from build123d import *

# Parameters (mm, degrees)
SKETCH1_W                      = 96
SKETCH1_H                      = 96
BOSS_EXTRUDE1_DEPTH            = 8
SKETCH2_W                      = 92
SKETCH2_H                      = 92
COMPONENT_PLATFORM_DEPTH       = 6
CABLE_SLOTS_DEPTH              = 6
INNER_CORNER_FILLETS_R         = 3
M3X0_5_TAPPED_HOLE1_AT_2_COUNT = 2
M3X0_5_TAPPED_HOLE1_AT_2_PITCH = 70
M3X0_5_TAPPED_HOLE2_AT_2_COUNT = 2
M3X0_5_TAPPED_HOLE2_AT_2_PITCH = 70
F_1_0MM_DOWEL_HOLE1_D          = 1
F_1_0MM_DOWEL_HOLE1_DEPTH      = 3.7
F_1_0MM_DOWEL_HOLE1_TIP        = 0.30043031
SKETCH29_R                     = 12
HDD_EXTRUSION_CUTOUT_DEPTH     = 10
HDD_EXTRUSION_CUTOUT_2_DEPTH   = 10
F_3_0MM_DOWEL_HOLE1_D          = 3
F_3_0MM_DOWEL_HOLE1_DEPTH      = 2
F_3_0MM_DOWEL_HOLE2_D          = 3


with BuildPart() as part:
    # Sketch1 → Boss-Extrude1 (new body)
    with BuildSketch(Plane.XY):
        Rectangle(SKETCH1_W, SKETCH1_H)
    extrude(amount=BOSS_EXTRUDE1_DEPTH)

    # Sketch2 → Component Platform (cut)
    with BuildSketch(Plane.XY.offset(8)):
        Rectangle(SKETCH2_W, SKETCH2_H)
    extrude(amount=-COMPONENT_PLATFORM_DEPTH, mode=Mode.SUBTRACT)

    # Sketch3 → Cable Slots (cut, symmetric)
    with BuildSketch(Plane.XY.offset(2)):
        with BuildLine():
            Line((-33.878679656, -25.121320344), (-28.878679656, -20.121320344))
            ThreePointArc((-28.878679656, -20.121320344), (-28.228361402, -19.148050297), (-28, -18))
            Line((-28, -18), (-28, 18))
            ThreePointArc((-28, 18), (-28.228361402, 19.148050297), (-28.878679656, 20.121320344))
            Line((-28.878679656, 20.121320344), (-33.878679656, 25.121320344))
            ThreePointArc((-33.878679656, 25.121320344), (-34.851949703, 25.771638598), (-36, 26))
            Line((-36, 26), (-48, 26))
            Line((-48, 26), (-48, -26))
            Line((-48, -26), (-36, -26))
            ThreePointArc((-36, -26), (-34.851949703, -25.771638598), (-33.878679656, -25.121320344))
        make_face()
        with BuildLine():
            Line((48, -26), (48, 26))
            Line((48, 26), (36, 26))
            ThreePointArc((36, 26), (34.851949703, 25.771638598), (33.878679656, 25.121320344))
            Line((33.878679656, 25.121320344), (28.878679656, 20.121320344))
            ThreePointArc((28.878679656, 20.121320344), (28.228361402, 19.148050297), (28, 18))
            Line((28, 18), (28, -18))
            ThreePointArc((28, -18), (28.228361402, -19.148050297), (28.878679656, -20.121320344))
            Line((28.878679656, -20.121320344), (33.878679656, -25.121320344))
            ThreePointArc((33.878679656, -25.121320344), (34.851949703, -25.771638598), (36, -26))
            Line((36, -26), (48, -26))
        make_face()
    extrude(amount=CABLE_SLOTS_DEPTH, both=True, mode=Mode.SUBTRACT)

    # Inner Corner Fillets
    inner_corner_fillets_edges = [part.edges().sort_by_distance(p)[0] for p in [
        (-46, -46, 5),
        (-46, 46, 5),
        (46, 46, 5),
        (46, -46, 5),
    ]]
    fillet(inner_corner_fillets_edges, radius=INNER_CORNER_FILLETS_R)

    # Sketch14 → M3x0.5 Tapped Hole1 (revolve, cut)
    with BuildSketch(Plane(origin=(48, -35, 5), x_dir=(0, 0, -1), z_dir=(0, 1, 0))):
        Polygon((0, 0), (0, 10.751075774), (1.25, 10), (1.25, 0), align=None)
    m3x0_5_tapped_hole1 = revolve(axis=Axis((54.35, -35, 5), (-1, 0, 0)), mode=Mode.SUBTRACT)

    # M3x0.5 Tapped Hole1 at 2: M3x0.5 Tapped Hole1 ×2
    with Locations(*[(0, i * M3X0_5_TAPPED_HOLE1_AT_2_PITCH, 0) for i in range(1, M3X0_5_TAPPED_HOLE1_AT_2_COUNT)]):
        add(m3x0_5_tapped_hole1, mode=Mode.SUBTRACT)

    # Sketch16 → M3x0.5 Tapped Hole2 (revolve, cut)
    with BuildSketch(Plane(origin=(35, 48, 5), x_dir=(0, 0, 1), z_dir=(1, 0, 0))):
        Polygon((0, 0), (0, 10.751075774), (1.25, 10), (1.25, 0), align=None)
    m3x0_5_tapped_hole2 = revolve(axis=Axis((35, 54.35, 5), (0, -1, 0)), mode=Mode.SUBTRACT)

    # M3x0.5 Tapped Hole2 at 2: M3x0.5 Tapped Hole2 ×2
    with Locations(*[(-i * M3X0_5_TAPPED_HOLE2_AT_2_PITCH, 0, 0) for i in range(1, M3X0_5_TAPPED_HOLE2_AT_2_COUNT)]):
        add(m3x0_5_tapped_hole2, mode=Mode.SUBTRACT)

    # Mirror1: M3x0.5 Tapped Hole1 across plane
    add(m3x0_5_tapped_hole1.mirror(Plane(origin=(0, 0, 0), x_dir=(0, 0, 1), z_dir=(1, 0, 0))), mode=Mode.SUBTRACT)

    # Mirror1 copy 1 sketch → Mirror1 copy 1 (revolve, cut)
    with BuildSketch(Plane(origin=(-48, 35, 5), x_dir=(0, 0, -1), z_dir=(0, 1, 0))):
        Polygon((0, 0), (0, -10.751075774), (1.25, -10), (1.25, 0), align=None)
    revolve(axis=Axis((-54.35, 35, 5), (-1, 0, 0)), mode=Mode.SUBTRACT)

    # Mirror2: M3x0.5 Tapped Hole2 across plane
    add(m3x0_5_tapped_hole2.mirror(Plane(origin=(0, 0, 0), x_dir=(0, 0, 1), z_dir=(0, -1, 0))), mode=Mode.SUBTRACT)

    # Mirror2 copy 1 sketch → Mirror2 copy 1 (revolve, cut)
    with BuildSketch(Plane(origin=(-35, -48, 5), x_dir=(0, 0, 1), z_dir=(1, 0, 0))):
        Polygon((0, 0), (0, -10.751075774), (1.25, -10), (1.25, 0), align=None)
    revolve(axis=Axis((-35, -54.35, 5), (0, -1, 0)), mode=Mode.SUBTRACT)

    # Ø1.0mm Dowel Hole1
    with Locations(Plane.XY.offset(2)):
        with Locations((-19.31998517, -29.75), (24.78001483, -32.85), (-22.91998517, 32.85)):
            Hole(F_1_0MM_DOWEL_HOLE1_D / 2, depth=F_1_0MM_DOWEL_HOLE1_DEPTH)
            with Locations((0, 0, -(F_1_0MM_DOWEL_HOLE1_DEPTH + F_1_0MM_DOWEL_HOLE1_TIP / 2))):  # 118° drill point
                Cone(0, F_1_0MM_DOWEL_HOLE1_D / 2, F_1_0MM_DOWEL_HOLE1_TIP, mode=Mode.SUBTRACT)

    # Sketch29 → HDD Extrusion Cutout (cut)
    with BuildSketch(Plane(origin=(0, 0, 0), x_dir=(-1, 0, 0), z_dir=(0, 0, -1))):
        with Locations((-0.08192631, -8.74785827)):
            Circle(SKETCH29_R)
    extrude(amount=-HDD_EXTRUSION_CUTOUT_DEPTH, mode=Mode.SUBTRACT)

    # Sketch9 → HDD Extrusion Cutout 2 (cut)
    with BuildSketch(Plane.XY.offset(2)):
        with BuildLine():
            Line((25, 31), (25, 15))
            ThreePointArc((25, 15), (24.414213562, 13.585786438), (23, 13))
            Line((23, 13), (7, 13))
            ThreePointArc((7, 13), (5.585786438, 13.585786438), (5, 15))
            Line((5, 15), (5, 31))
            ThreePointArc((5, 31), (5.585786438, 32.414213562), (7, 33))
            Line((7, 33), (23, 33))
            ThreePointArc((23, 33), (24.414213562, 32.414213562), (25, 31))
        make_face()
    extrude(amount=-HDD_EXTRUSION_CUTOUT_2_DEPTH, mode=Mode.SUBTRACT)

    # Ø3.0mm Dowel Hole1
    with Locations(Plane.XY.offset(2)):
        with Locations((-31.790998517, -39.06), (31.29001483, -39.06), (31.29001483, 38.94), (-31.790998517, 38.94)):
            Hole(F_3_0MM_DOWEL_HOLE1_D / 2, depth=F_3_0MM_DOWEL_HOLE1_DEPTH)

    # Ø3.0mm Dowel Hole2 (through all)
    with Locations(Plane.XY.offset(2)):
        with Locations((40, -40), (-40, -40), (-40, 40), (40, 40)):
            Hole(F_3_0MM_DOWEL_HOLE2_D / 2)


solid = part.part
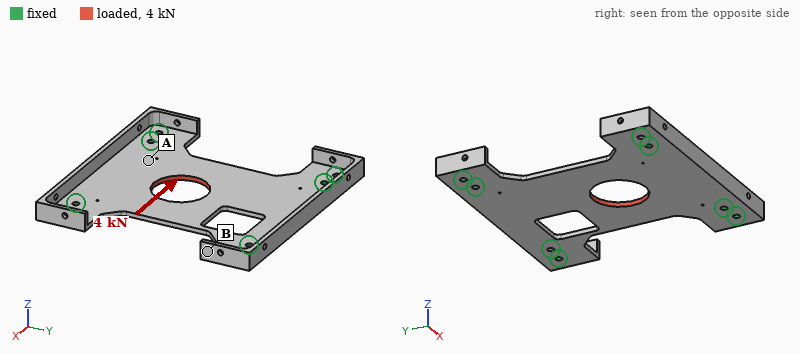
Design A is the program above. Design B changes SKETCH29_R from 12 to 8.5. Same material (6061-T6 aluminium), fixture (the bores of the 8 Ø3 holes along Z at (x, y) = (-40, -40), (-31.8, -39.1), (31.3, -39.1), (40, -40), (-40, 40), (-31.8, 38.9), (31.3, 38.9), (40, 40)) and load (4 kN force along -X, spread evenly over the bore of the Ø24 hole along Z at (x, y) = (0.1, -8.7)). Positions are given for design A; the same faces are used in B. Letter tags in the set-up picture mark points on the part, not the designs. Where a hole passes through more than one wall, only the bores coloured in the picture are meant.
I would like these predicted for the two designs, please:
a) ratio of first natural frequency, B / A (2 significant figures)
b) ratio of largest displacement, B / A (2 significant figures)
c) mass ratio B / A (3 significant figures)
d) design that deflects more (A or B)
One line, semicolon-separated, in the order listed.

0.98; 0.92; 1.03; A
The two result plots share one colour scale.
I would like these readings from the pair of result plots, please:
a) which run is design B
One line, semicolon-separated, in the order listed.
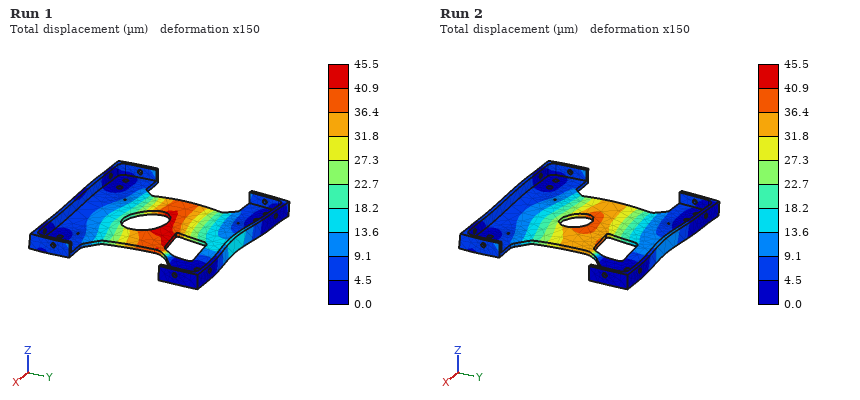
Run 2
